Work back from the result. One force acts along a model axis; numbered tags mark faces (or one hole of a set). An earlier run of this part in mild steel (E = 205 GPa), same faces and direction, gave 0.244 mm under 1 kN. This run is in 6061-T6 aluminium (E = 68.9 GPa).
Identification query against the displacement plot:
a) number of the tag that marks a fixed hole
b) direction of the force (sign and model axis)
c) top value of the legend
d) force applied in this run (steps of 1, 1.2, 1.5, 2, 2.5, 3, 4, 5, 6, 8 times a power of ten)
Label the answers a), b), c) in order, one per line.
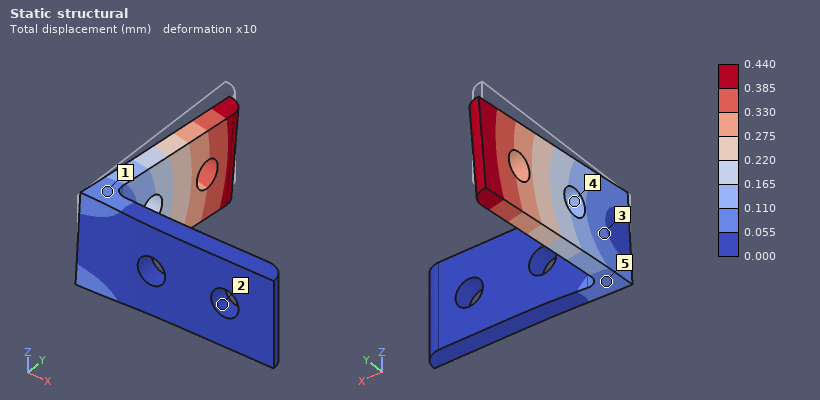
a) 2
b) -Z
c) 0.440 mm
d) 600 N
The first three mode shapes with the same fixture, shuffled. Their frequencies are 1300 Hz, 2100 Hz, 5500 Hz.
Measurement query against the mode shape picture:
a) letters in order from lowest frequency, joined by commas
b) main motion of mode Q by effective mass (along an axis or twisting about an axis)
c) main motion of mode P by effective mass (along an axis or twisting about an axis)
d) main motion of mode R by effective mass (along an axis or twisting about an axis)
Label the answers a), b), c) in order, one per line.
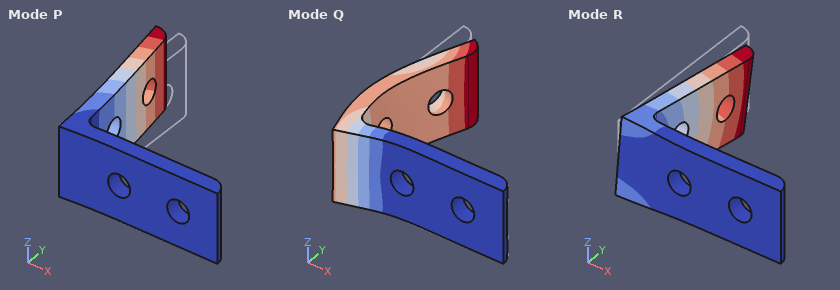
a) P, R, Q
b) along Y
c) along X
d) along Z
